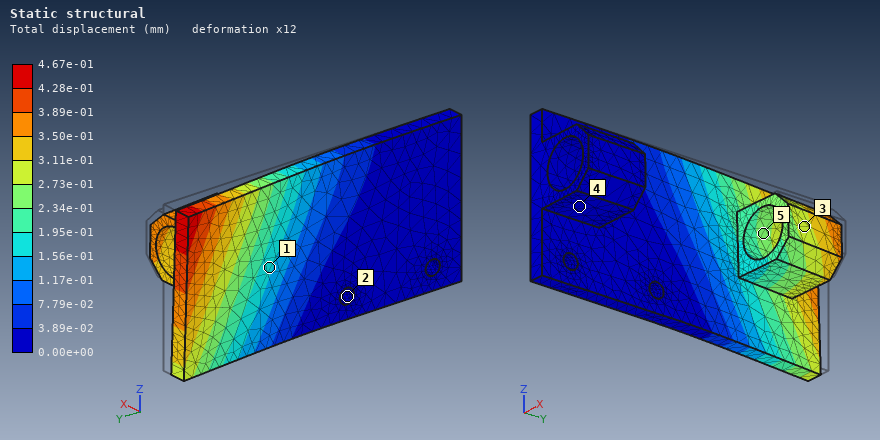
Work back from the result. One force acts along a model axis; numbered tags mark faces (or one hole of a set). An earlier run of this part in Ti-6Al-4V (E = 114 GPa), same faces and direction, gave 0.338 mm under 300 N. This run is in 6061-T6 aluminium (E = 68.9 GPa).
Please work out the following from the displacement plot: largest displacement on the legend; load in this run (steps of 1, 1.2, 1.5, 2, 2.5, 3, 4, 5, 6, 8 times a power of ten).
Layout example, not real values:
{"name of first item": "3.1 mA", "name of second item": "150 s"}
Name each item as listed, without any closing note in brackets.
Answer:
{"largest displacement on the legend": "4.67e-01 mm", "load in this run": "250 N"}
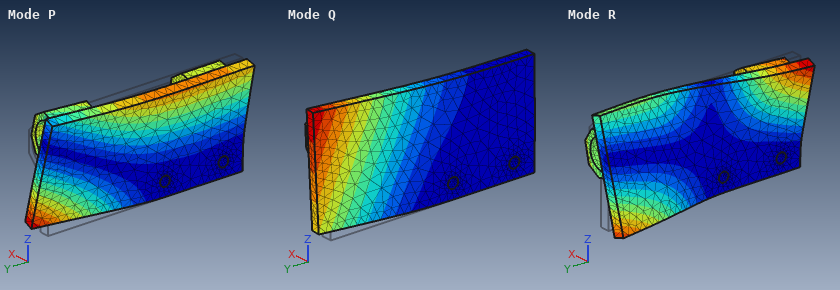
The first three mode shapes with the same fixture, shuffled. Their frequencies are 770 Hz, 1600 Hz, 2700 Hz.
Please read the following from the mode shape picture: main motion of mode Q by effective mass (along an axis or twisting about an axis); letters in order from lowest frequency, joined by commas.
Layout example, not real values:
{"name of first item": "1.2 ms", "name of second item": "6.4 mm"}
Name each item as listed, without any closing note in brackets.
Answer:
{"main motion of mode Q by effective mass": "along X", "letters in order from lowest frequency, joined by commas": "Q, P, R"}
